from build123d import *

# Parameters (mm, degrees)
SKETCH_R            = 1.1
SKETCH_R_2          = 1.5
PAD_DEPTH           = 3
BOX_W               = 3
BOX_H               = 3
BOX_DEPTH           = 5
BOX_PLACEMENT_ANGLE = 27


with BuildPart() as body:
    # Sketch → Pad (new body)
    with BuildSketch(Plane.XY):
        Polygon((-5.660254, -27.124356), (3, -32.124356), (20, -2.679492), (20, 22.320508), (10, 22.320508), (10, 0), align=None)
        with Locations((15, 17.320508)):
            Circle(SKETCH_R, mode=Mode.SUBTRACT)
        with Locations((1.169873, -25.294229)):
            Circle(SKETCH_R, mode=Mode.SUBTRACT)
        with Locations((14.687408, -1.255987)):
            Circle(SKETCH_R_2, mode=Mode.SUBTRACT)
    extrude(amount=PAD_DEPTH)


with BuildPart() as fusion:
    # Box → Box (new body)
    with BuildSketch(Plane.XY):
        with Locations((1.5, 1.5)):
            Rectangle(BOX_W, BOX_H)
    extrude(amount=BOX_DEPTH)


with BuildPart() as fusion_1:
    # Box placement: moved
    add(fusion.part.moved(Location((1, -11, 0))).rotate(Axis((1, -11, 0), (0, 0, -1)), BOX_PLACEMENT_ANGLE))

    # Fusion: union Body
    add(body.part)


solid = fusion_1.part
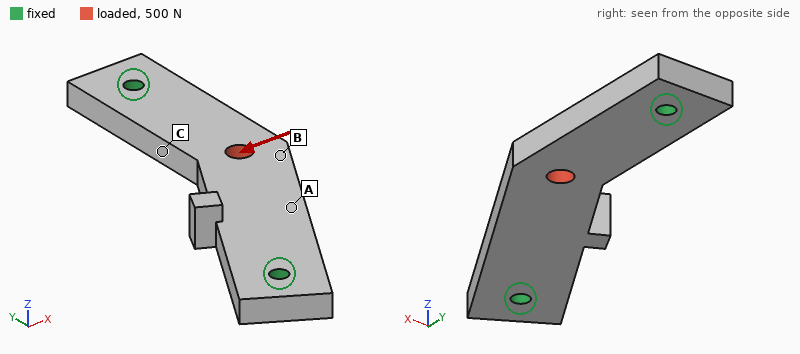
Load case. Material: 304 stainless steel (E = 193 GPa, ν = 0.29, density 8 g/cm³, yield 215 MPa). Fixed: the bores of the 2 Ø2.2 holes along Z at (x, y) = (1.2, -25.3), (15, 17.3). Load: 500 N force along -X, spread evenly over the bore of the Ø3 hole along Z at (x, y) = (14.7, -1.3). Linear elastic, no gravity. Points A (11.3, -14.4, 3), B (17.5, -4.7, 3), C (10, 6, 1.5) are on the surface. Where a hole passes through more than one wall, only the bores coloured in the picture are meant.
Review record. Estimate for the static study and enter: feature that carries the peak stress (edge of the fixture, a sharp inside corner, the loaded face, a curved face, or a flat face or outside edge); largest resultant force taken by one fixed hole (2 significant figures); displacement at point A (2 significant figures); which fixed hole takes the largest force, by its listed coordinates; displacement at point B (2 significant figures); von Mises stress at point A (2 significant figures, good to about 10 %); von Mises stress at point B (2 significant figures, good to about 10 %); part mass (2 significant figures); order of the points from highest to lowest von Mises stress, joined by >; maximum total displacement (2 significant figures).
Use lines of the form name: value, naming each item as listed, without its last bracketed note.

feature that carries the peak stress: edge of the fixture
largest resultant force taken by one fixed hole: 470 N
displacement at point A: 5.0 µm
which fixed hole takes the largest force, by its listed coordinates: (1.2, -25.3)
displacement at point B: 7.5 µm
von Mises stress at point A: 24 MPa
von Mises stress at point B: 44 MPa
part mass: 13 g
order of the points from highest to lowest von Mises stress, joined by >: B > A > C
maximum total displacement: 8.1 µm
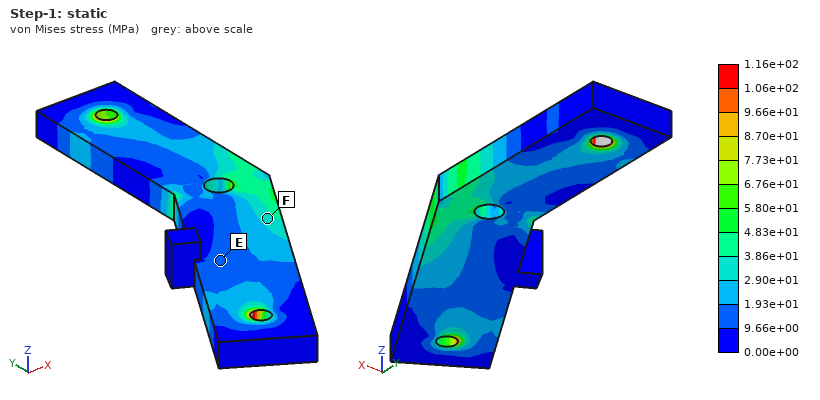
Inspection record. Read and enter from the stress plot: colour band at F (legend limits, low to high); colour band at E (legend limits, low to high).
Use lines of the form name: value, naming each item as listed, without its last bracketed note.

colour band at F: 2.90e+01 to 3.86e+01 MPa
colour band at E: 9.66e+00 to 1.93e+01 MPa
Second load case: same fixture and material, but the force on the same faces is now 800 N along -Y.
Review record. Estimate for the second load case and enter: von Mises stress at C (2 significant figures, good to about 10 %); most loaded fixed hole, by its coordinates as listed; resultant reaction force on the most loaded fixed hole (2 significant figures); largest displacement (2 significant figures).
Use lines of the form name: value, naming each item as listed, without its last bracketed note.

von Mises stress at C: 17 MPa
most loaded fixed hole, by its coordinates as listed: (15, 17.3)
resultant reaction force on the most loaded fixed hole: 630 N
largest displacement: 3.7 µm
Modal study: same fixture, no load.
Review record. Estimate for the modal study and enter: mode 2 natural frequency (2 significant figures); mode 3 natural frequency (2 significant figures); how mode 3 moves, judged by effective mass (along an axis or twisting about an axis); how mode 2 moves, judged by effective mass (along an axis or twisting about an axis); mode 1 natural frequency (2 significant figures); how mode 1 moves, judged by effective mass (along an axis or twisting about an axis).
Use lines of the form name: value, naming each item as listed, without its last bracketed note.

mode 2 natural frequency: 15 kHz
mode 3 natural frequency: 17 kHz
how mode 3 moves, judged by effective mass: along X
how mode 2 moves, judged by effective mass: twisting about Y
mode 1 natural frequency: 6500 Hz
how mode 1 moves, judged by effective mass: along Z
